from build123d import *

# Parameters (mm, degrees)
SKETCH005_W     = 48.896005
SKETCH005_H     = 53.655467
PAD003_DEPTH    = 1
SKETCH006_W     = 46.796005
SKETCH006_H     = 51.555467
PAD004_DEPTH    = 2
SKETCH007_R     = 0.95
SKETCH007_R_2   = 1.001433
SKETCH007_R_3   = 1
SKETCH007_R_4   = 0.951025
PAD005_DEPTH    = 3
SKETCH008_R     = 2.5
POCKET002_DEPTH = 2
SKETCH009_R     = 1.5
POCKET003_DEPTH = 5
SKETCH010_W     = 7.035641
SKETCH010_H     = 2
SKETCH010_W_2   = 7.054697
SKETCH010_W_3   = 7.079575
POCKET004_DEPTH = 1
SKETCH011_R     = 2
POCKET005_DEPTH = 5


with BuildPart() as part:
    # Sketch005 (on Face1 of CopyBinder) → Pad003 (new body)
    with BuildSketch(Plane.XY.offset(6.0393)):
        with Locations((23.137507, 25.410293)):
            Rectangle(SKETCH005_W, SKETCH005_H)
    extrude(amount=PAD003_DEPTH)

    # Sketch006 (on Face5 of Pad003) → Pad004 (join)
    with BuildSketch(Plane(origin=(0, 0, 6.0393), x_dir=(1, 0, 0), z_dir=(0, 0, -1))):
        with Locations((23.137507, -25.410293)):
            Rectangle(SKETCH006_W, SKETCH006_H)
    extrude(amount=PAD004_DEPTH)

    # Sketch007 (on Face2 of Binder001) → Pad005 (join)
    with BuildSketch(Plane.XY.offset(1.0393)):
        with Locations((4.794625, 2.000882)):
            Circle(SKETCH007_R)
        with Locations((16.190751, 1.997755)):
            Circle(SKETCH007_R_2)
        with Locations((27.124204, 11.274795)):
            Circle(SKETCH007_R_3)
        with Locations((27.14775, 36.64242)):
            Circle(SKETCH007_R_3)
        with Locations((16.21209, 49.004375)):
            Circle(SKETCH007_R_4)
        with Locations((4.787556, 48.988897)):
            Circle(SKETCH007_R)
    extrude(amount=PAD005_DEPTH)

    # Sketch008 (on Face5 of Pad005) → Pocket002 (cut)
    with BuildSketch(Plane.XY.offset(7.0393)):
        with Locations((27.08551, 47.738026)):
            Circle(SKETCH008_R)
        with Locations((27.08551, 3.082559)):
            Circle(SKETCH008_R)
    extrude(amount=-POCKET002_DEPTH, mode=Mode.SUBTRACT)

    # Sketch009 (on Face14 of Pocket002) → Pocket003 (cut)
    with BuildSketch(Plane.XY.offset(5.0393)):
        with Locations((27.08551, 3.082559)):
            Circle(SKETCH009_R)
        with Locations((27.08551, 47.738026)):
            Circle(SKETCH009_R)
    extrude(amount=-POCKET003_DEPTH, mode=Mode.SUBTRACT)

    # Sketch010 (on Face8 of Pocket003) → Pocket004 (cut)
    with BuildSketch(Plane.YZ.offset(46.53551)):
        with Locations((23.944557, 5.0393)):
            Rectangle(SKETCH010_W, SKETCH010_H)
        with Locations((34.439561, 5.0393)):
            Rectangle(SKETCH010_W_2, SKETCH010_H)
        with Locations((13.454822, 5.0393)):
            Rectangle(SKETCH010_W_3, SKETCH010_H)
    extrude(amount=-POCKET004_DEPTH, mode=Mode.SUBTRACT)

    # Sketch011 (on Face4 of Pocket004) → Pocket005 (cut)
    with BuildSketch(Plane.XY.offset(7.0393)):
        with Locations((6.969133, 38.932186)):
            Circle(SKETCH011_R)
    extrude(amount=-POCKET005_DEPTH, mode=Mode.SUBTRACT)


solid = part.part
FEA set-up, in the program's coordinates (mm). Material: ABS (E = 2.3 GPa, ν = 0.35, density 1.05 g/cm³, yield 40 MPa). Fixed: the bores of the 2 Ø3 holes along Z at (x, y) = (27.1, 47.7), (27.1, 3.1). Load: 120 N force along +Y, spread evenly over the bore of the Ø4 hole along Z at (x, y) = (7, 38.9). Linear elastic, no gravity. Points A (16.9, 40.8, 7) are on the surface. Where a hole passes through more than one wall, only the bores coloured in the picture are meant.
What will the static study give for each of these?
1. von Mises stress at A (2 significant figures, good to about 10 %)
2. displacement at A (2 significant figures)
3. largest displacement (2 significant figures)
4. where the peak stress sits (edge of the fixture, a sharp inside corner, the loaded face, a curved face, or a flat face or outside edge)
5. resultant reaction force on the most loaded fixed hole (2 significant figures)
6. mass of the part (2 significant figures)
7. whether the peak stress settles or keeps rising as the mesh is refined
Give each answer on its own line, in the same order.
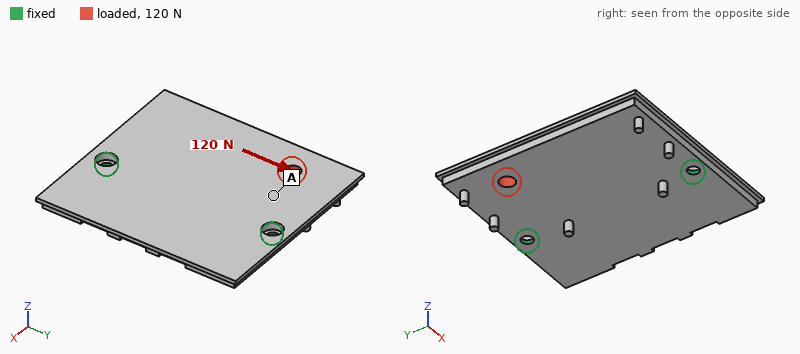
1.3 MPa
37 µm
92 µm
edge of the fixture
81 N
7.7 g
keeps rising
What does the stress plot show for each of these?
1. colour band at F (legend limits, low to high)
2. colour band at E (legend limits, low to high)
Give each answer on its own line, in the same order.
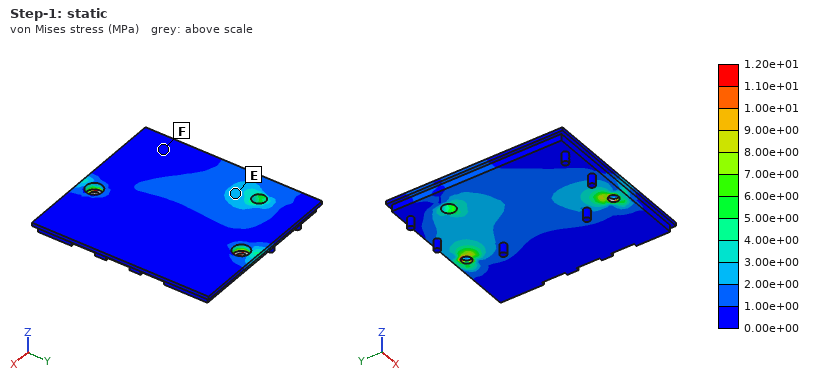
0.00e+00 to 1.00e+00 MPa
2.00e+00 to 3.00e+00 MPa
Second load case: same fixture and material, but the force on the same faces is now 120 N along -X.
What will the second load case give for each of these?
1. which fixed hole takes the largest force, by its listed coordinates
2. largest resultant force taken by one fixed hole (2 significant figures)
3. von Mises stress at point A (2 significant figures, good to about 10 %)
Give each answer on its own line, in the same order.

(27.1, 47.7)
96 N
1.9 MPa
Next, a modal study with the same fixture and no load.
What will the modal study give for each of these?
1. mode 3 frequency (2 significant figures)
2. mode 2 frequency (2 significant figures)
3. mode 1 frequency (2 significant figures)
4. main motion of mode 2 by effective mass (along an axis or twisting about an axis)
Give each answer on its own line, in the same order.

1200 Hz
1000 Hz
420 Hz
along Z
